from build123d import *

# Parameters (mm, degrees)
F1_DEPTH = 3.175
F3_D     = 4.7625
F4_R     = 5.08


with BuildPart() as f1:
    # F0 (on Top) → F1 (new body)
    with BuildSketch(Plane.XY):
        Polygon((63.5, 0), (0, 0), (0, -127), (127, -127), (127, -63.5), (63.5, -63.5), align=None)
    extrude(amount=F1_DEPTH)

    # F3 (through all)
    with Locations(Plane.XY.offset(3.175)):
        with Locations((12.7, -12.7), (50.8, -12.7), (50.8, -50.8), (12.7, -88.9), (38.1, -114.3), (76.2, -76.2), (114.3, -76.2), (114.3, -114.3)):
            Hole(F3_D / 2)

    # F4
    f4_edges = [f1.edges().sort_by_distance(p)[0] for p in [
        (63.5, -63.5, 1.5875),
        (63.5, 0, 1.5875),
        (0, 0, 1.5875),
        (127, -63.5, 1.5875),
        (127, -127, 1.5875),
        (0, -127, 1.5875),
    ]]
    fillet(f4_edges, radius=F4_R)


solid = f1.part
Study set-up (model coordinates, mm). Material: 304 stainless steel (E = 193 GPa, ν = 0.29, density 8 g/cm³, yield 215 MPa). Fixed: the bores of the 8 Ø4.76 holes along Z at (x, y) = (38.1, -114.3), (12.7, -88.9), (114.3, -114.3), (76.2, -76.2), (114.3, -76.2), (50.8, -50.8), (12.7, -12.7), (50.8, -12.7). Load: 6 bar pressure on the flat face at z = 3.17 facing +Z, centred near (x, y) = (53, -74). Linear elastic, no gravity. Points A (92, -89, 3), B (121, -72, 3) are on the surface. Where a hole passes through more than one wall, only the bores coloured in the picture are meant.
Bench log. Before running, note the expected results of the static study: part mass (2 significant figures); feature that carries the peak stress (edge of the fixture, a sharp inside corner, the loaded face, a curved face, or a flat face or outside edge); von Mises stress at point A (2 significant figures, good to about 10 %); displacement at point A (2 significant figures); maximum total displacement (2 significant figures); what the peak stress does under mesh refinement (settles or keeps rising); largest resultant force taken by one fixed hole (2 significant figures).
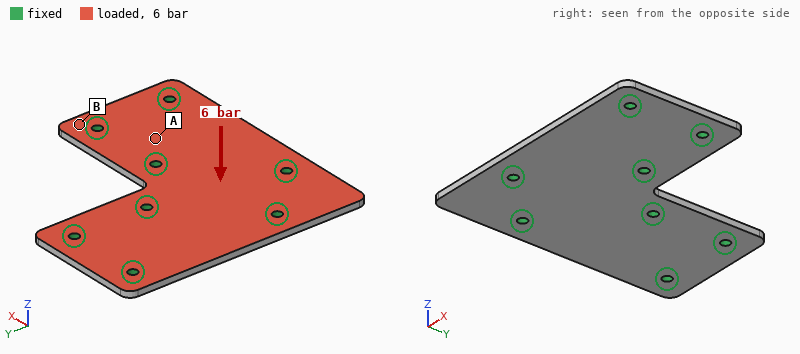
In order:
300 g
edge of the fixture
38 MPa
22 µm
97 µm
keeps rising
1.2 kN
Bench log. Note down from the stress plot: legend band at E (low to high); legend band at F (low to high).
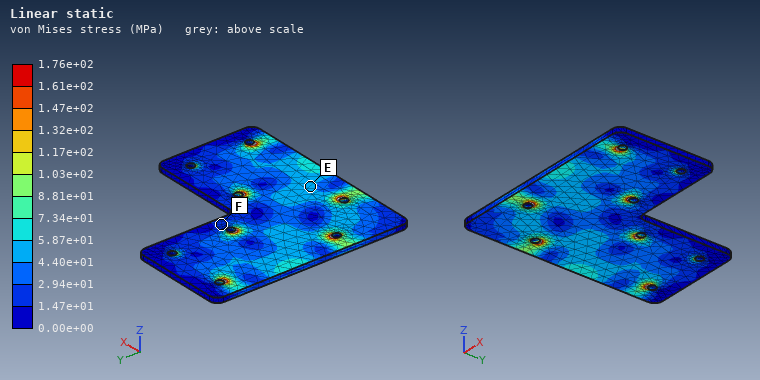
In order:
4.40e+01 to 5.87e+01 MPa
1.47e+01 to 2.94e+01 MPa
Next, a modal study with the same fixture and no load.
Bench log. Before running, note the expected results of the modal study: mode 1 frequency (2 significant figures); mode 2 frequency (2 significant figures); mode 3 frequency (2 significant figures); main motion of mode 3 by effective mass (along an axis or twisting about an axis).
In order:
3200 Hz
3200 Hz
3400 Hz
along Z
